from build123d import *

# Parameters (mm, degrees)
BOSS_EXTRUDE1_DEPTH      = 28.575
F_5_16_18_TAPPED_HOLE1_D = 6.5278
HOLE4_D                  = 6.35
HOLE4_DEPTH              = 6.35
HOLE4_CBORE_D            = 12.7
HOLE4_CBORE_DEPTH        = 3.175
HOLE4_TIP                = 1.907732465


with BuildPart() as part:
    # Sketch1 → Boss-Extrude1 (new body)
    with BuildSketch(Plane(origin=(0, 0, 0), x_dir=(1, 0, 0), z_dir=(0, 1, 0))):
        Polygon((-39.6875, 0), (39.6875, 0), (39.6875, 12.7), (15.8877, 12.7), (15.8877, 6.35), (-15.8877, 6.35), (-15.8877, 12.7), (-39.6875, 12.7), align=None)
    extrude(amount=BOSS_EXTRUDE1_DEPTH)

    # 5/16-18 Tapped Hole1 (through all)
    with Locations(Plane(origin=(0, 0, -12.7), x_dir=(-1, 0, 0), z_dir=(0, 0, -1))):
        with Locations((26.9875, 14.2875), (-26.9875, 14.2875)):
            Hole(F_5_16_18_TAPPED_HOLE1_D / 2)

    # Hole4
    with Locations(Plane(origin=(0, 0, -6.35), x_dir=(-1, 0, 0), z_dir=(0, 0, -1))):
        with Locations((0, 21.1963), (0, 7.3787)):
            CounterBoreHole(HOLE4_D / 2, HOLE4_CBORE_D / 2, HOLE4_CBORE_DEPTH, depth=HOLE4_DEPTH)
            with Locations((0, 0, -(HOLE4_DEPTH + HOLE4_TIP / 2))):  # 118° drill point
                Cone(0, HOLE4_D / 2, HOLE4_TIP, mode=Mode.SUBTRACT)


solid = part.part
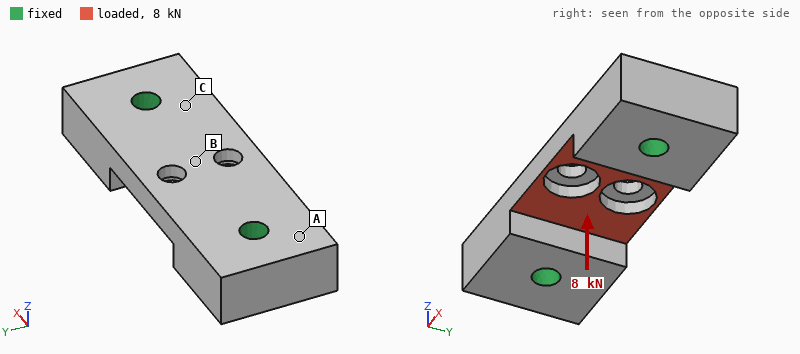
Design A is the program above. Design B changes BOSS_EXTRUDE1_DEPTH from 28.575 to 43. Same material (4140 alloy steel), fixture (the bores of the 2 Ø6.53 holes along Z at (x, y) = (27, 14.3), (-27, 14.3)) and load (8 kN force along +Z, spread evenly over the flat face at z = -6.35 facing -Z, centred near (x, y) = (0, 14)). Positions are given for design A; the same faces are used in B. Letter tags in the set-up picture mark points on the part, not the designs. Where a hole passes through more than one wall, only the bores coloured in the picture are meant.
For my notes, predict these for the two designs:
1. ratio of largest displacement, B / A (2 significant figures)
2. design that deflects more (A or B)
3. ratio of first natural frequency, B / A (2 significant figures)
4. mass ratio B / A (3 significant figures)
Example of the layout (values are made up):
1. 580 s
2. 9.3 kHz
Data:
1. 1.6
2. B
3. 0.53
4. 1.55
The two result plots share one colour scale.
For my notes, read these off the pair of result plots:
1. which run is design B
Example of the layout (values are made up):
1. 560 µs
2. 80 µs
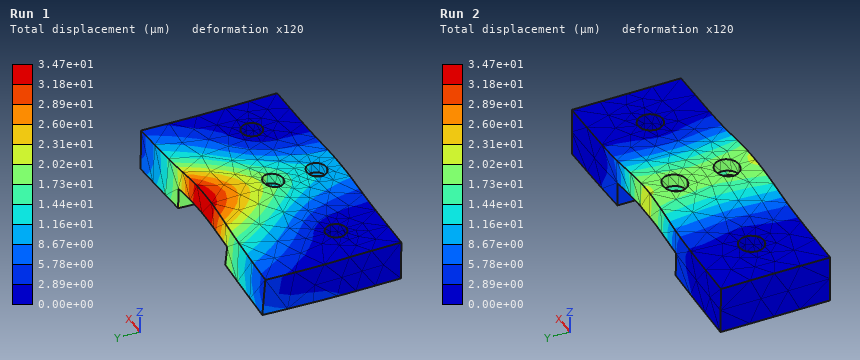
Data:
1. Run 1
